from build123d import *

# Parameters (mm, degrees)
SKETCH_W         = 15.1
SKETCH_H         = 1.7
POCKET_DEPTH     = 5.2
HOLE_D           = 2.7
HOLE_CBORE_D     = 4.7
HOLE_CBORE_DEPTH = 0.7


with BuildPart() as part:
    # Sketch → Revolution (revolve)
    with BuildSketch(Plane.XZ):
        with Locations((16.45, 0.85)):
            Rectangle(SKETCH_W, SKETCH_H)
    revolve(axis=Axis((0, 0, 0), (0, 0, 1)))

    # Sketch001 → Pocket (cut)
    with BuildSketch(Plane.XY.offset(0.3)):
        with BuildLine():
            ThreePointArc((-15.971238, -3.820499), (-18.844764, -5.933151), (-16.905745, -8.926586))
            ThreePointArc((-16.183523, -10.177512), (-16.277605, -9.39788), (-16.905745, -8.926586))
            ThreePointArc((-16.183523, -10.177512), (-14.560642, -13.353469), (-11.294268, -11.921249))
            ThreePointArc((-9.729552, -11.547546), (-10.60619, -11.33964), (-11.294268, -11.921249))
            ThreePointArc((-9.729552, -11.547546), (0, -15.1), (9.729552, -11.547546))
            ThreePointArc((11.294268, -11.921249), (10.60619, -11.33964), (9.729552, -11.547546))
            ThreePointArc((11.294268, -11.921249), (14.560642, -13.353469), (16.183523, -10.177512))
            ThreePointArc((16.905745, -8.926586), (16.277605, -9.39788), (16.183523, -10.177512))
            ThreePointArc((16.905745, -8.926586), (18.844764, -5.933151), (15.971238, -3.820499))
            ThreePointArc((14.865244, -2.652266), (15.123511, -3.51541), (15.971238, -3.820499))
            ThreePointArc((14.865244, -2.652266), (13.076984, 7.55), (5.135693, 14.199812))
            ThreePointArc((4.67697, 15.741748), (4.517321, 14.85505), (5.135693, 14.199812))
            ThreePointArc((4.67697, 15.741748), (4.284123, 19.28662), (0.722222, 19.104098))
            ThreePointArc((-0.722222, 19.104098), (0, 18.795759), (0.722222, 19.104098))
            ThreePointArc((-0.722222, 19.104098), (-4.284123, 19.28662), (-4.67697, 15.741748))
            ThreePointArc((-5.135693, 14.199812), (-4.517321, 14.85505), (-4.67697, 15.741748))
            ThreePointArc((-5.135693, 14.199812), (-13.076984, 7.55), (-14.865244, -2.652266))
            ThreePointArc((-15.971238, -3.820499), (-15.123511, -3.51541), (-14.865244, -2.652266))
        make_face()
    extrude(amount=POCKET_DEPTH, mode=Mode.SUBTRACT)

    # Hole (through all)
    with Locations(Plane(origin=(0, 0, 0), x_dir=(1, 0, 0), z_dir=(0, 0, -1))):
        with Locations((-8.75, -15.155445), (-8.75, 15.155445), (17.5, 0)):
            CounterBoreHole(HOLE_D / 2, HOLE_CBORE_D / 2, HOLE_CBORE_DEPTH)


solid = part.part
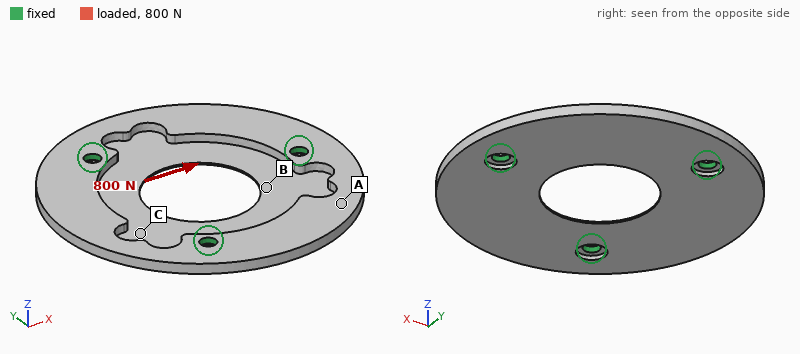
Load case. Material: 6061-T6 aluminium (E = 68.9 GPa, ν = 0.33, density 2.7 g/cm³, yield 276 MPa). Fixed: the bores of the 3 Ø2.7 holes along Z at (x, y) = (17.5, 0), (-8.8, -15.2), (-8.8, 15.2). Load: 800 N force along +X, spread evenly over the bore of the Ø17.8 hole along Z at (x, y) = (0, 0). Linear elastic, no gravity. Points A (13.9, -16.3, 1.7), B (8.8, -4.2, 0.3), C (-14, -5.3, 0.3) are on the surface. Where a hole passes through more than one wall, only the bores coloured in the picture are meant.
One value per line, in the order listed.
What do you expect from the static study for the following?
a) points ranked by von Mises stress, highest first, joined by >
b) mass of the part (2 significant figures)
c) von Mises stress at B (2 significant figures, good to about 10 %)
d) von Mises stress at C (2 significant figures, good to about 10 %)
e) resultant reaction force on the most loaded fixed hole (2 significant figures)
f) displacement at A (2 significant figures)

B > C > A
4.7 g
57 MPa
36 MPa
290 N
26 µm
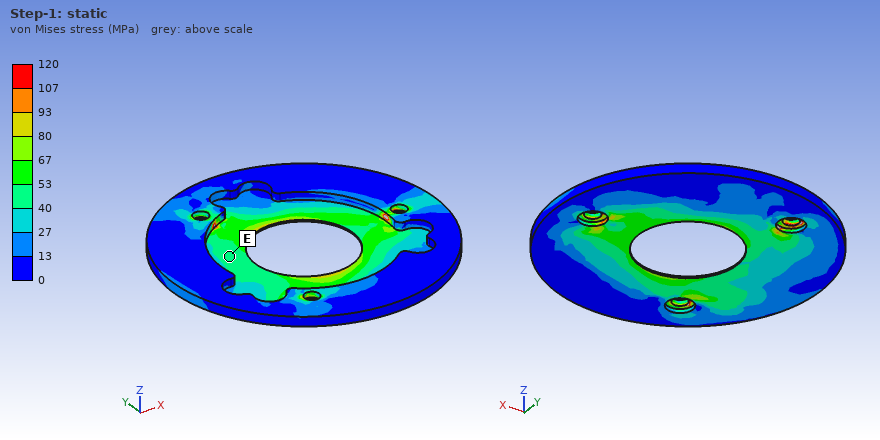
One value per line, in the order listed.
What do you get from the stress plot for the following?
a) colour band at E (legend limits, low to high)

40 to 53 MPa
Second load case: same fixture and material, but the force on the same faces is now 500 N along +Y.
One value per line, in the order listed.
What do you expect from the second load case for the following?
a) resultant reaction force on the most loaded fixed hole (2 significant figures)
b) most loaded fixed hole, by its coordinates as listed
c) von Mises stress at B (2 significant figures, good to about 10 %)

190 N
(17.5, 0)
42 MPa
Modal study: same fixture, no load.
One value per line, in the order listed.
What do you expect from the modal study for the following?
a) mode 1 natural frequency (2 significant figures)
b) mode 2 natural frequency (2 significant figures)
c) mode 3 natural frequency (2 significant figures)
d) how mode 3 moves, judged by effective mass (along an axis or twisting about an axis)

3700 Hz
3700 Hz
4300 Hz
along Z
